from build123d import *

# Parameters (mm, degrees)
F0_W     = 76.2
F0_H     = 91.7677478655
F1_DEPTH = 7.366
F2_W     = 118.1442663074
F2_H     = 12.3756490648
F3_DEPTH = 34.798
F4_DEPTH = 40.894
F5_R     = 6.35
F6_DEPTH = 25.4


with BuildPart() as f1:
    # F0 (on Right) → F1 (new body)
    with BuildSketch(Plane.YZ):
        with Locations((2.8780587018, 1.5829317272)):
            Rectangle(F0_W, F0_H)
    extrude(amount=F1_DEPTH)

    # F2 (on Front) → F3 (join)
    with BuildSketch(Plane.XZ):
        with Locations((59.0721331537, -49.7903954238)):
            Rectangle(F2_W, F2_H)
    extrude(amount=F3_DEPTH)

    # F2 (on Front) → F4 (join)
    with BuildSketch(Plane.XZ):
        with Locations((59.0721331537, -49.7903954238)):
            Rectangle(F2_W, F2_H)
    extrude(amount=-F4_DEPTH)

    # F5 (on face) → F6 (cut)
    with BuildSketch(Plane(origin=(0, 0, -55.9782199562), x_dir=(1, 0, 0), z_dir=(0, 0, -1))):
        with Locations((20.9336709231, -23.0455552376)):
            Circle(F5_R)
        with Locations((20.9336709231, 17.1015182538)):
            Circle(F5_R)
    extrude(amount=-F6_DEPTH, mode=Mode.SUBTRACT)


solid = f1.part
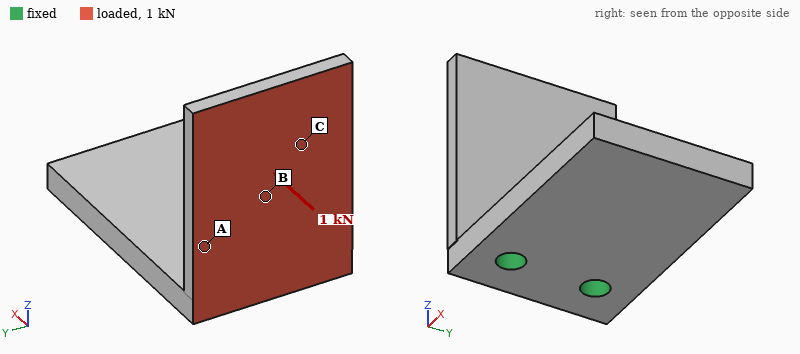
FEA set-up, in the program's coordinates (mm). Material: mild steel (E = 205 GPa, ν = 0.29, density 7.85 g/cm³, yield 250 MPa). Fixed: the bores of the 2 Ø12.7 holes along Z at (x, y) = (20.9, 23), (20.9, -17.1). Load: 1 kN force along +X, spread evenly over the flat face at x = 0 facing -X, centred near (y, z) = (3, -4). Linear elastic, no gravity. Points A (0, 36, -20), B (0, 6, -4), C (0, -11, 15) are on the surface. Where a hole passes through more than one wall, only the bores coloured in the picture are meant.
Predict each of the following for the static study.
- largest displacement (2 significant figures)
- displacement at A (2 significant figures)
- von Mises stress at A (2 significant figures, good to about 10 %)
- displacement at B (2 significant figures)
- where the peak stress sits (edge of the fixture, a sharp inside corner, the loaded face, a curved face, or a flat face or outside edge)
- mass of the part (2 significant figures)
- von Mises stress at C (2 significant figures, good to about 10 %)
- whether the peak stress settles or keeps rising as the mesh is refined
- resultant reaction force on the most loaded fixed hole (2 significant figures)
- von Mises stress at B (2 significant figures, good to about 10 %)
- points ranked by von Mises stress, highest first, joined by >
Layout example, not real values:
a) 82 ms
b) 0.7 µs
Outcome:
a) 0.20 mm
b) 0.031 mm
c) 32 MPa
d) 0.065 mm
e) a sharp inside corner
f) 1.2 kg
g) 7.5 MPa
h) keeps rising
i) 520 N
j) 17 MPa
k) A > B > C
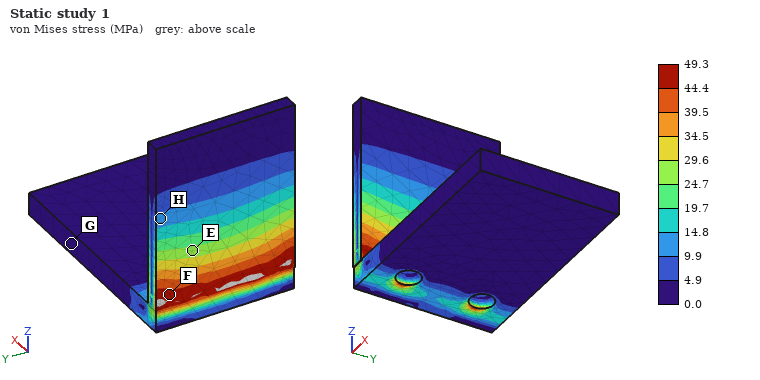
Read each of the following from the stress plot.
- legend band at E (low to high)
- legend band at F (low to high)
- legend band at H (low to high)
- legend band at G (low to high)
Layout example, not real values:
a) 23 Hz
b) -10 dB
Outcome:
a) 24.7 to 29.6 MPa
b) 44.4 to 49.3 MPa
c) 9.9 to 14.8 MPa
d) 0.0 to 4.9 MPa
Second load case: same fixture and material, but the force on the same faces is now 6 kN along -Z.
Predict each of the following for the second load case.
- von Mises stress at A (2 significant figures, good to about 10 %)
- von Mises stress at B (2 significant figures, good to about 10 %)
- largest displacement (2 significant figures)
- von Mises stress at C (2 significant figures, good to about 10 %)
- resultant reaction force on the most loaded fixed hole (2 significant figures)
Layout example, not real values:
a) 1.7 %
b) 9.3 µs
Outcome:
a) 28 MPa
b) 20 MPa
c) 0.15 mm
d) 13 MPa
e) 3.0 kN
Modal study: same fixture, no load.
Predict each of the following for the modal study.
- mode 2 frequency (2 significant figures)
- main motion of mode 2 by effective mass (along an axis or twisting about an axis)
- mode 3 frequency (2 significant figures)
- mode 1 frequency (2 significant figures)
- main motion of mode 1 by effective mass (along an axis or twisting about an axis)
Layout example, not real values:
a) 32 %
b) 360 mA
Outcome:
a) 1100 Hz
b) along Z
c) 1900 Hz
d) 650 Hz
e) along X
